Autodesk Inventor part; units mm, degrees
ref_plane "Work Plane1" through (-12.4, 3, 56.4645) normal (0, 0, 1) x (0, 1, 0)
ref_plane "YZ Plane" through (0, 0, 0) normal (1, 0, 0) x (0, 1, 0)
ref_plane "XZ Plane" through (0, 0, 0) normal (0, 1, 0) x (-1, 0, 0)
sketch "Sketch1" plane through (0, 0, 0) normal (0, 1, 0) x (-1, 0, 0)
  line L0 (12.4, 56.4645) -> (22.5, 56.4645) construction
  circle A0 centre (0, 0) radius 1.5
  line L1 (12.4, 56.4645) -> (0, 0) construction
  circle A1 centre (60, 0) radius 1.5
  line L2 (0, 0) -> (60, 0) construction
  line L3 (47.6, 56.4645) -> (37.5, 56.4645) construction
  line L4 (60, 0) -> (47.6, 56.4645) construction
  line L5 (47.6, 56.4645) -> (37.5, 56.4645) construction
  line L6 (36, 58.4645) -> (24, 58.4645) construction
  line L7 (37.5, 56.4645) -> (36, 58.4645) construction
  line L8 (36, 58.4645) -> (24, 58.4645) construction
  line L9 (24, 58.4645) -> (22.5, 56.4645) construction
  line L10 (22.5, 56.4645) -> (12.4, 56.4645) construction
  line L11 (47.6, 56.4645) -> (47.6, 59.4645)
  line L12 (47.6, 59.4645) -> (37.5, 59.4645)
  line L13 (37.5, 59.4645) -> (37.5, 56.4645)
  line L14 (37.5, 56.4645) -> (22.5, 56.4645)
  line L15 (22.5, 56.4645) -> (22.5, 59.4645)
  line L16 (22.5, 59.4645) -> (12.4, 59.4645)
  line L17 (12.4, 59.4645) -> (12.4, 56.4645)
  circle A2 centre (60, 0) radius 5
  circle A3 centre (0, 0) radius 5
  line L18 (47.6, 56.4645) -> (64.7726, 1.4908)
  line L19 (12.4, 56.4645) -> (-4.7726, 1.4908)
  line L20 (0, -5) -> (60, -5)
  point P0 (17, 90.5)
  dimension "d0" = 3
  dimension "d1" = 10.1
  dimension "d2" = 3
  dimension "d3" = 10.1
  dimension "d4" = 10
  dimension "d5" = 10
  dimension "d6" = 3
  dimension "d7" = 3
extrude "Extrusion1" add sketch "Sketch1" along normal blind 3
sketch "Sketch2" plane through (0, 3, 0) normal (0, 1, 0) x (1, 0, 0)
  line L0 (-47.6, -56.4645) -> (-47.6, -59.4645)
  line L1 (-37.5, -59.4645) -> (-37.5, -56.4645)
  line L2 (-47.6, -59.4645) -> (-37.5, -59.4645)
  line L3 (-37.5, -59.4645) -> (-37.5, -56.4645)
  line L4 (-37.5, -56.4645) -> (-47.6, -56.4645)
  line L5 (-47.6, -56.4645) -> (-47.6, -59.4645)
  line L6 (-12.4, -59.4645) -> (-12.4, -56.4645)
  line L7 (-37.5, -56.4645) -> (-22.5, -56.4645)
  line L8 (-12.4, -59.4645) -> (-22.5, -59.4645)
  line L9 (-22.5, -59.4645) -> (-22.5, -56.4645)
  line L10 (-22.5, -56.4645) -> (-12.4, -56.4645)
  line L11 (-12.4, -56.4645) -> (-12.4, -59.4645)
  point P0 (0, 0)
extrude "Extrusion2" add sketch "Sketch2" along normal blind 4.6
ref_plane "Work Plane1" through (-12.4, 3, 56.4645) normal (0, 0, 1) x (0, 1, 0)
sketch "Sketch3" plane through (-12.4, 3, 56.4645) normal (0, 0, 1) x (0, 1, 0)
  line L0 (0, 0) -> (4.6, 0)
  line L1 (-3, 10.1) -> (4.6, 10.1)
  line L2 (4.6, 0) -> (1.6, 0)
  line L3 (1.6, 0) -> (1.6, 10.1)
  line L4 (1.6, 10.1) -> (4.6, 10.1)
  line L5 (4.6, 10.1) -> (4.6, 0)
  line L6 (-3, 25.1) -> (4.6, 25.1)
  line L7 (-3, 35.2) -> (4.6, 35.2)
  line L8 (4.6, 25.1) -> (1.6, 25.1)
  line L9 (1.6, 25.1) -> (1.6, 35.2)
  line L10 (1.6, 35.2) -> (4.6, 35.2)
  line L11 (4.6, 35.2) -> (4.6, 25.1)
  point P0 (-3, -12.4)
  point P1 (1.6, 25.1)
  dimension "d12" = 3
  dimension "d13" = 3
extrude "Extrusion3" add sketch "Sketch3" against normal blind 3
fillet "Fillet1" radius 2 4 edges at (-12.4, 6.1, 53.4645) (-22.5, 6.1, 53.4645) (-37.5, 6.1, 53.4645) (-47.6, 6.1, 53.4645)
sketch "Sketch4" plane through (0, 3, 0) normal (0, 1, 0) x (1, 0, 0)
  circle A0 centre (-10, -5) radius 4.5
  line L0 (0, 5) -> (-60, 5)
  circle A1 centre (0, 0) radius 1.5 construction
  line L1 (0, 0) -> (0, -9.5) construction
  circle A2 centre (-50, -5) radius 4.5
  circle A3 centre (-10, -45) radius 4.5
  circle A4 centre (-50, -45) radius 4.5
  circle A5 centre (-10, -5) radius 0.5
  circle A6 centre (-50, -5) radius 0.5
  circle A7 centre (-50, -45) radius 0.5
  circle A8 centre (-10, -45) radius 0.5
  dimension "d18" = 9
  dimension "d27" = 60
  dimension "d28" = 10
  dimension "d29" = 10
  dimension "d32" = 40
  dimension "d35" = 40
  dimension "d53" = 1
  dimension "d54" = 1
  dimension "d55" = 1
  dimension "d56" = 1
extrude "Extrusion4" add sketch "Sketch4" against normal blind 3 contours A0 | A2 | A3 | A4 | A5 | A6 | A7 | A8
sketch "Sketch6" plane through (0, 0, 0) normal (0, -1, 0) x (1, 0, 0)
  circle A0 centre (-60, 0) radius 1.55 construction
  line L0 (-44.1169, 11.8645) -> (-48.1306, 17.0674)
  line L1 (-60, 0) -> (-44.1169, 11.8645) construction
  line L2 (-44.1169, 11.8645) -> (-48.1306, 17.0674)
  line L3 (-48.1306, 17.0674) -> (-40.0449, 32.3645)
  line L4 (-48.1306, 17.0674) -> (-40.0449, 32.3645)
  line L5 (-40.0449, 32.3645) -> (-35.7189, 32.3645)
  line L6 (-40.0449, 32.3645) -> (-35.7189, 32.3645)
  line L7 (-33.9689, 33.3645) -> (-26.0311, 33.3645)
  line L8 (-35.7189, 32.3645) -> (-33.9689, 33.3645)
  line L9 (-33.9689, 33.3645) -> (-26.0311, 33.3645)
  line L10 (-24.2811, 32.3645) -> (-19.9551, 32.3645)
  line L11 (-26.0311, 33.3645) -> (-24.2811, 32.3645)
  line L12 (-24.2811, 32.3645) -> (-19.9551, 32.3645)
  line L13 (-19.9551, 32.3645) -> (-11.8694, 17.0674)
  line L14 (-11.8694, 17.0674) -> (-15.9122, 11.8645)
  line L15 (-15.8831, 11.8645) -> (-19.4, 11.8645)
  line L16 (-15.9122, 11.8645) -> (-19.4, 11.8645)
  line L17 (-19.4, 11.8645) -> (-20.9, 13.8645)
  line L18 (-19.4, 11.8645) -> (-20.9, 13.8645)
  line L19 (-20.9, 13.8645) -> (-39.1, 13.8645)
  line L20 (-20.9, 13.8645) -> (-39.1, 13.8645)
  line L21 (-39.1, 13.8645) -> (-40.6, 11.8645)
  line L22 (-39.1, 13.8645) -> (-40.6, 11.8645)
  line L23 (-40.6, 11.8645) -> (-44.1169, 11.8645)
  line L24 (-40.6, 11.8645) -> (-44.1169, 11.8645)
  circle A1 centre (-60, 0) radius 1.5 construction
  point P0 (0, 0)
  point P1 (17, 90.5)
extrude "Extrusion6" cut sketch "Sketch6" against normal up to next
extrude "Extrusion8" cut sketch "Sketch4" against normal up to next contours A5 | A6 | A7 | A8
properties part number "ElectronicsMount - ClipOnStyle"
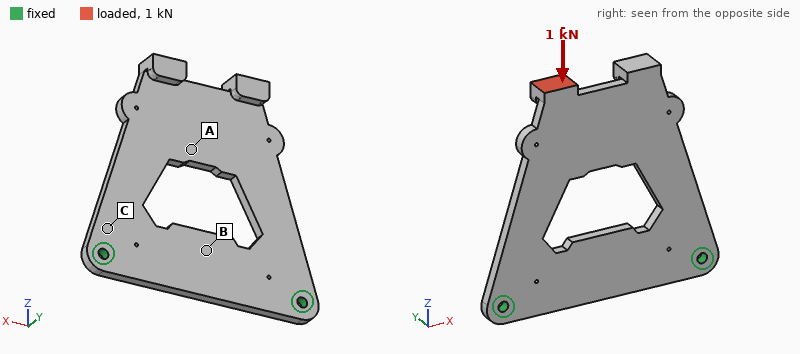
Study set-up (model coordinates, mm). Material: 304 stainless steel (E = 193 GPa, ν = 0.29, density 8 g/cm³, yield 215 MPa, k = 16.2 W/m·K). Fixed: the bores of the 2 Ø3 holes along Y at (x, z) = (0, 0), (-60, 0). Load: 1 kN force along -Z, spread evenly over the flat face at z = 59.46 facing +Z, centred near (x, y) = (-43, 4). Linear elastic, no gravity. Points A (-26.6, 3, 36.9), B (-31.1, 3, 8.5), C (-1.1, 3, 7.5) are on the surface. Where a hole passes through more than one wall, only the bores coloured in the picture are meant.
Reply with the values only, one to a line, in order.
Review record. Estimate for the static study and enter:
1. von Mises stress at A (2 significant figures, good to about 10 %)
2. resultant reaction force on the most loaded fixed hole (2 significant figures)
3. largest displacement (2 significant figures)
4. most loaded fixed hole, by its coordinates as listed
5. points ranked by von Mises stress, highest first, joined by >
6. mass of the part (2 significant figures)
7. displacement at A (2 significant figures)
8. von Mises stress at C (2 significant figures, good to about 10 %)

32 MPa
730 N
0.37 mm
(-60, 0)
C > A > B
72 g
0.13 mm
54 MPa
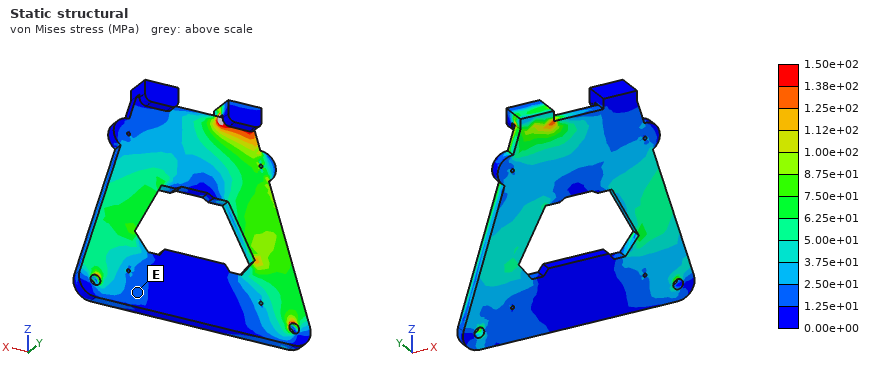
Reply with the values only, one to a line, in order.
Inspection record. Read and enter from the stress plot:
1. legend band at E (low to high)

1.25e+01 to 2.50e+01 MPa
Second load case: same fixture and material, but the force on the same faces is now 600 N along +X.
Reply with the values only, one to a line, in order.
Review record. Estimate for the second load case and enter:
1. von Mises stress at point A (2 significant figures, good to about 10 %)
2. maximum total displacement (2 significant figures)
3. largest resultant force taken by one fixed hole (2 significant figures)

31 MPa
53 µm
660 N
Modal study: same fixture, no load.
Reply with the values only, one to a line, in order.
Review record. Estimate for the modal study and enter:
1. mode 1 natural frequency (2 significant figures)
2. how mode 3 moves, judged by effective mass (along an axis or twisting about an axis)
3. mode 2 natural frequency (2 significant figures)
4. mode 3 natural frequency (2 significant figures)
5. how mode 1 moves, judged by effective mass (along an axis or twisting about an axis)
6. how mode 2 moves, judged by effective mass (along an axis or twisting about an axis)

520 Hz
along Y
1900 Hz
3100 Hz
along Y
twisting about Z
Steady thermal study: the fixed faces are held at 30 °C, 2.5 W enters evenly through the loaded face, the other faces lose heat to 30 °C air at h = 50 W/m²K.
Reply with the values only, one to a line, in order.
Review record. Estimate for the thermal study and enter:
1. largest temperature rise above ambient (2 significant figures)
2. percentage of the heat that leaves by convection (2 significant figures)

53 K
95 %
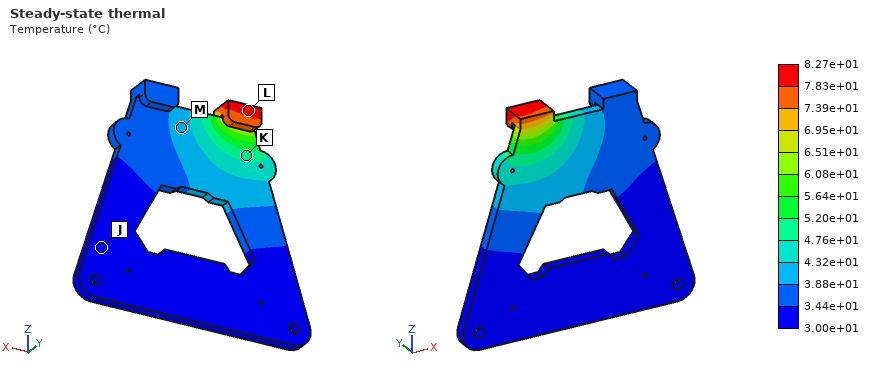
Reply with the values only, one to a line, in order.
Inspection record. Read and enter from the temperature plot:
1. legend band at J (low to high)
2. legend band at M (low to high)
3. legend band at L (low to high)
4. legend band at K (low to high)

3.00e+01 to 3.44e+01 °C
3.88e+01 to 4.32e+01 °C
7.83e+01 to 8.27e+01 °C
4.76e+01 to 5.20e+01 °C
